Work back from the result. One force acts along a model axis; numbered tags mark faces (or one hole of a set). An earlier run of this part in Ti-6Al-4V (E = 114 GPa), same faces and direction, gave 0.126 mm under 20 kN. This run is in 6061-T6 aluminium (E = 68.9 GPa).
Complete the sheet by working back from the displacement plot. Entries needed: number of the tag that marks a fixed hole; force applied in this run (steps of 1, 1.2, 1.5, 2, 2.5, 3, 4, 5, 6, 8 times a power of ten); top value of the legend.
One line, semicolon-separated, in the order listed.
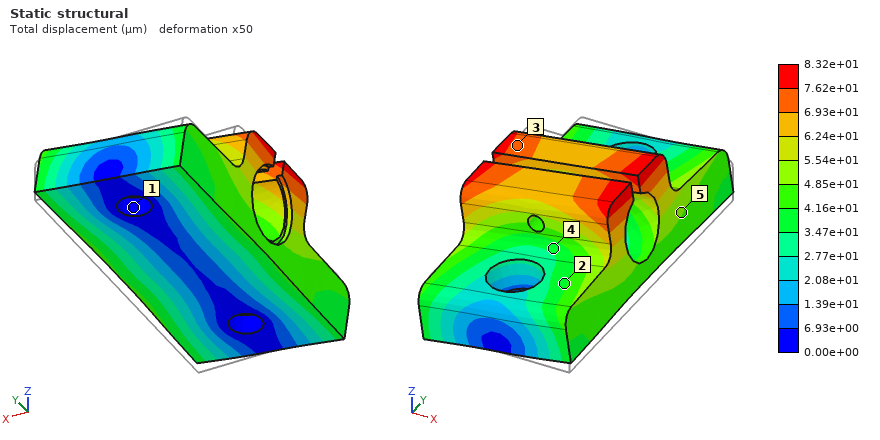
1; 8 kN; 8.32e+01 µm
